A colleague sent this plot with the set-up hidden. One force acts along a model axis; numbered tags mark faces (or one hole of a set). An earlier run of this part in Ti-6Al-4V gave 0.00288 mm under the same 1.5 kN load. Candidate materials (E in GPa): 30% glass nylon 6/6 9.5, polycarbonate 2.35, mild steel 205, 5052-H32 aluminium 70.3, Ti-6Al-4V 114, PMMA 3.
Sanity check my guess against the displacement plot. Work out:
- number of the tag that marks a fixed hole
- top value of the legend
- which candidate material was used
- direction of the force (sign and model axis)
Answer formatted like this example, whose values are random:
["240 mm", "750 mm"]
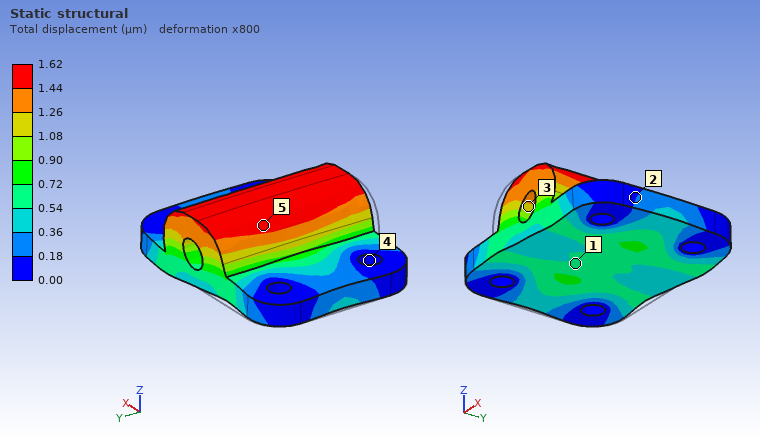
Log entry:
["4", "1.62 µm", "mild steel", "+X"]
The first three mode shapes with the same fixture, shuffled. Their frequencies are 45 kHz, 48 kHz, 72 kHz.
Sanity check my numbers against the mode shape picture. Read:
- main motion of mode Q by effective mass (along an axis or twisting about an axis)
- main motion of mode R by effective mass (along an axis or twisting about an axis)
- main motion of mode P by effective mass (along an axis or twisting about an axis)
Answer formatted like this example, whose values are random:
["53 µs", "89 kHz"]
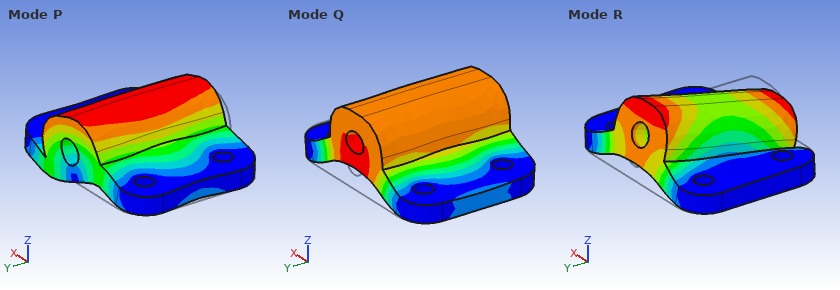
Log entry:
["along Z", "along Y", "along X"]
